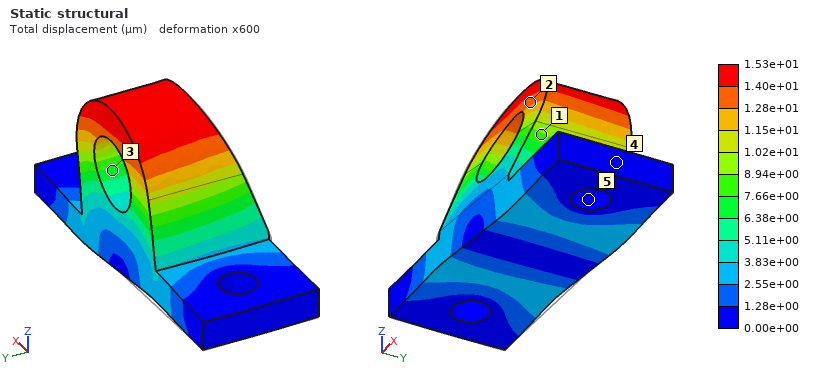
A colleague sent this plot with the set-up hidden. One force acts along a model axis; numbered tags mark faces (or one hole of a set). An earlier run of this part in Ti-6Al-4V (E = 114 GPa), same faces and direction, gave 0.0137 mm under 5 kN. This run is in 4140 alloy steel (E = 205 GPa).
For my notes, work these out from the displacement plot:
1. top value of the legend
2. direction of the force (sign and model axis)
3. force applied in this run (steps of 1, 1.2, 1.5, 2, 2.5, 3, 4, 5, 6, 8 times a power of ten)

1.53e+01 µm
+X
10 kN
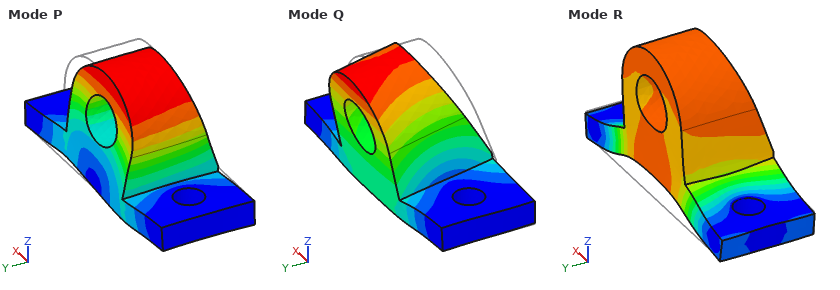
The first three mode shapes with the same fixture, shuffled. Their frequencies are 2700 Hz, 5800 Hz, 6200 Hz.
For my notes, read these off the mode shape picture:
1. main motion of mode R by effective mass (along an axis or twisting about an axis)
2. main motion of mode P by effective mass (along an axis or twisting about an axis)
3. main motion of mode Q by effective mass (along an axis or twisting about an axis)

along Z
along X
along Y
